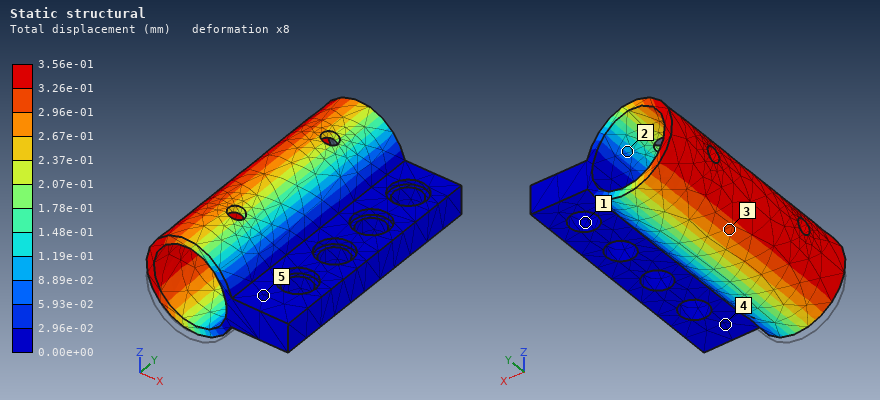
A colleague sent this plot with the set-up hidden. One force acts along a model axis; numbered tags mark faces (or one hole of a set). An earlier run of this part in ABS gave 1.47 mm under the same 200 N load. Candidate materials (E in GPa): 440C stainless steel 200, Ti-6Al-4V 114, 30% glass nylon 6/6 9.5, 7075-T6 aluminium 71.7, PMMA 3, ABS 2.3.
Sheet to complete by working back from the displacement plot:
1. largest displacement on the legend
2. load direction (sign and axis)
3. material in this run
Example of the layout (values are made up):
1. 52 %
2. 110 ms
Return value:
1. 3.56e-01 mm
2. +Z
3. 30% glass nylon 6/6
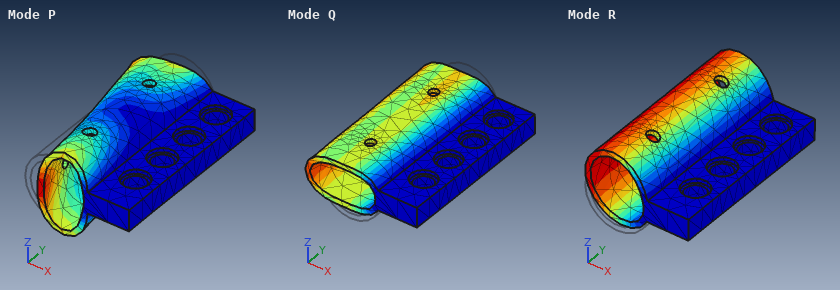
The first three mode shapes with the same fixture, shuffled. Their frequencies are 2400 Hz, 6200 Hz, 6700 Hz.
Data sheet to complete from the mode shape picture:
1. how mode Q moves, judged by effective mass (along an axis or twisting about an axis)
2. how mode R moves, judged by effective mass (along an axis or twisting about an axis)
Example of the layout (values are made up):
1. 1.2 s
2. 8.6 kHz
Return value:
1. along X
2. along Z
